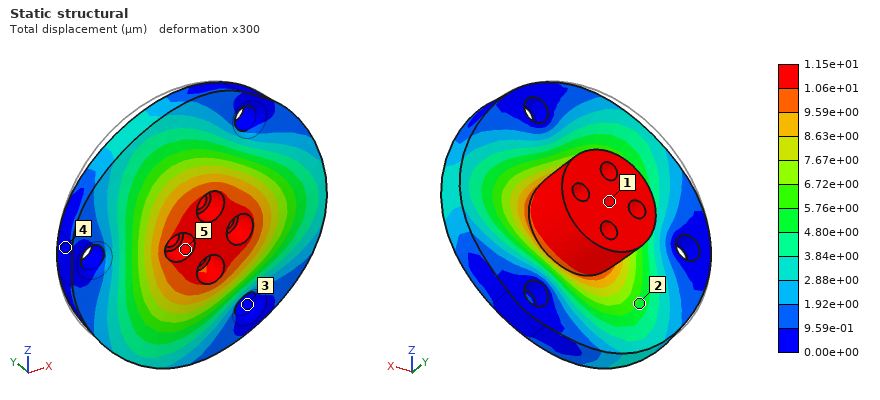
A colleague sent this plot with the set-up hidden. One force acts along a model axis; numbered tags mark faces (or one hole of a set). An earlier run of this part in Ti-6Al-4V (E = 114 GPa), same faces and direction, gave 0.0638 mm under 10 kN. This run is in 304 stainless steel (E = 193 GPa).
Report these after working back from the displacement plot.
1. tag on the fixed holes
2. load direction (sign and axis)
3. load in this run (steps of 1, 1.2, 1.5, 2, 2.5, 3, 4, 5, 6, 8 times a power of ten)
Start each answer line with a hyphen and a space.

- 3
- -Y
- 3 kN
